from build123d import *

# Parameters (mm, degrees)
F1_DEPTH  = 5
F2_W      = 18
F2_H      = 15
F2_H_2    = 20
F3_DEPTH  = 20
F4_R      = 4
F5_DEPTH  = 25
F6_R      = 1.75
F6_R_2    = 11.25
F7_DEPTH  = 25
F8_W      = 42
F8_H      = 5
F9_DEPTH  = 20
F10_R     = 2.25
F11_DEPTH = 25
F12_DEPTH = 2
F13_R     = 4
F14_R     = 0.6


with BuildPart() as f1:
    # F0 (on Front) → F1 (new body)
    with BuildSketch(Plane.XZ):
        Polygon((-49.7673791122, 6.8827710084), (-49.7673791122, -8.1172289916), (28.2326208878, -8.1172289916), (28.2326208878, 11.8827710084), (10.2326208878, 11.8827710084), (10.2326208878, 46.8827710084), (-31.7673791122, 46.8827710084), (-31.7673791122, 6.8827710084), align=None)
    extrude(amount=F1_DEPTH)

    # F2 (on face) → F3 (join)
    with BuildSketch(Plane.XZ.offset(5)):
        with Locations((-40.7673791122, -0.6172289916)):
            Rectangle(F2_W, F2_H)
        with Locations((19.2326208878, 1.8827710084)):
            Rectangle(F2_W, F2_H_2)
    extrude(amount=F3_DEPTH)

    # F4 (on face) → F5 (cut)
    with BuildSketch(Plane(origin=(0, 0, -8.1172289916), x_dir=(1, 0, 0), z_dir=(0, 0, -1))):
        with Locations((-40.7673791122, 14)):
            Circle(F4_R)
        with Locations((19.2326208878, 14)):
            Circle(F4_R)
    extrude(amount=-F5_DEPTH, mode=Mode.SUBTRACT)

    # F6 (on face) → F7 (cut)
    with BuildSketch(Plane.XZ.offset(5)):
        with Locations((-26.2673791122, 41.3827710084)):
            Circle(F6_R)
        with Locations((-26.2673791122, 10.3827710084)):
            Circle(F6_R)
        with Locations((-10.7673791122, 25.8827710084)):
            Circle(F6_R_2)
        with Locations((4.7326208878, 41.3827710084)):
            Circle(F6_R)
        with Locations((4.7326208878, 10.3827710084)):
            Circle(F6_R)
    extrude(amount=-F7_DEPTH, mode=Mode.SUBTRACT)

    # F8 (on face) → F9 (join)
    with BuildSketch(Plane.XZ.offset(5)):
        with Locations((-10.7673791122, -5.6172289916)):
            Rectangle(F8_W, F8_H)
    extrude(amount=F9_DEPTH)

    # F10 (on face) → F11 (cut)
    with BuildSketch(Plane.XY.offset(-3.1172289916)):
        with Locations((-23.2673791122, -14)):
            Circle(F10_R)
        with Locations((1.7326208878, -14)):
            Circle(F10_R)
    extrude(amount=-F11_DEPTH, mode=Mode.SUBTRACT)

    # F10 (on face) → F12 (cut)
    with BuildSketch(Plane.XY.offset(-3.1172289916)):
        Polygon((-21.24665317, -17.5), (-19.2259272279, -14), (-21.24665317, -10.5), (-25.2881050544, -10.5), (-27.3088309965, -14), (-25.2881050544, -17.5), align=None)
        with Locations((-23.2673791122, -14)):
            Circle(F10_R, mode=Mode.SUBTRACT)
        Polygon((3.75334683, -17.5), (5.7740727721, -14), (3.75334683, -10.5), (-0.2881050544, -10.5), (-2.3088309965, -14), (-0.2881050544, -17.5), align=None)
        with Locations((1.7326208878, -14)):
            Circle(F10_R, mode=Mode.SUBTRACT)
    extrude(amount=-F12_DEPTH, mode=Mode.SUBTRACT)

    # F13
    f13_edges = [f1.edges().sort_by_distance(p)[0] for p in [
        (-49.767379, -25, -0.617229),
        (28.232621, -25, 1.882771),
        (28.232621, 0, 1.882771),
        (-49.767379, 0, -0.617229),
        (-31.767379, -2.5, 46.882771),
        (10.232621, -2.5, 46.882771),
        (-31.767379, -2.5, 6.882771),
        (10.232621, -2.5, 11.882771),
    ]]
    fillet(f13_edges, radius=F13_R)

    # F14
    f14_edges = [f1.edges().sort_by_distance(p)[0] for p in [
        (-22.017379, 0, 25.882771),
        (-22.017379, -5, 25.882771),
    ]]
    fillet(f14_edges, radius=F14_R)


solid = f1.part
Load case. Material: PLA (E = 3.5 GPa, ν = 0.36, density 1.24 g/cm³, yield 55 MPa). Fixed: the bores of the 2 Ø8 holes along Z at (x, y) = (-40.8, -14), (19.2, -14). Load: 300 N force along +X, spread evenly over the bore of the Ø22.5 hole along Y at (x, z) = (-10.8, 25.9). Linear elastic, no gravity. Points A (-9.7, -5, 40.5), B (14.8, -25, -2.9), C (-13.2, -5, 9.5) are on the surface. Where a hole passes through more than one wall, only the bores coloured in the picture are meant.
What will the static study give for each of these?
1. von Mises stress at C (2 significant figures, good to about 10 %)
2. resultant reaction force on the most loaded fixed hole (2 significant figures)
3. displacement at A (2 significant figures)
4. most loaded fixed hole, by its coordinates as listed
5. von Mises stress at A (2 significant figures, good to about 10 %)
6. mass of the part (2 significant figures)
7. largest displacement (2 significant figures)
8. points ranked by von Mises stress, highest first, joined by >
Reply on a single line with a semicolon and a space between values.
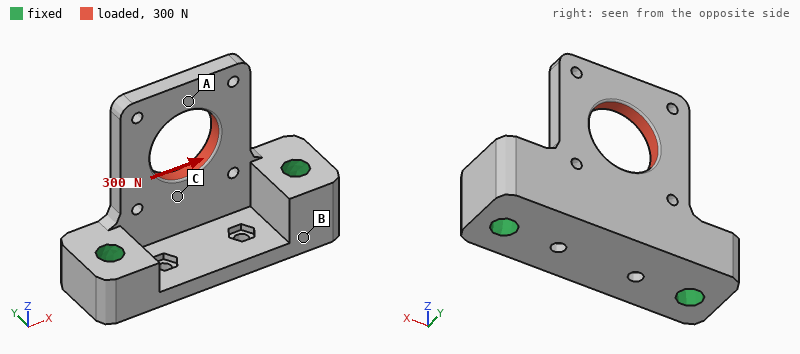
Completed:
3.7 MPa; 230 N; 0.13 mm; (19.2, -14); 2.1 MPa; 34 g; 0.15 mm; C > A > B
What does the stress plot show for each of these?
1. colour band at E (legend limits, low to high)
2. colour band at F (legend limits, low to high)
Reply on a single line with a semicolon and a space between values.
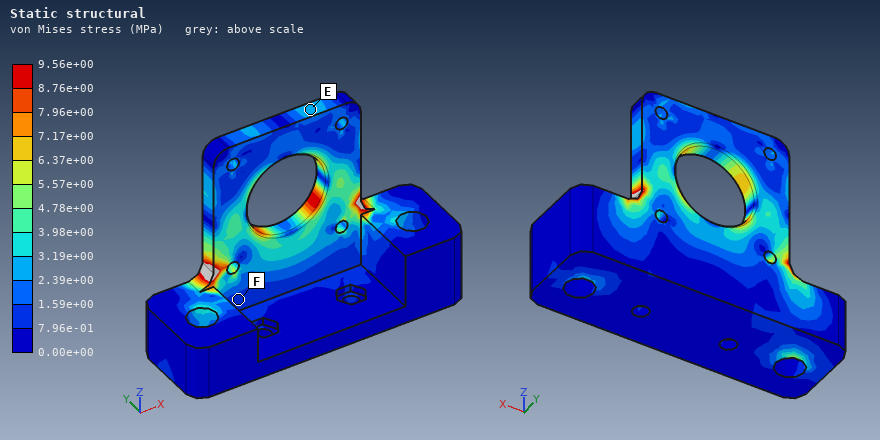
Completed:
2.39e+00 to 3.19e+00 MPa; 7.96e-01 to 1.59e+00 MPa
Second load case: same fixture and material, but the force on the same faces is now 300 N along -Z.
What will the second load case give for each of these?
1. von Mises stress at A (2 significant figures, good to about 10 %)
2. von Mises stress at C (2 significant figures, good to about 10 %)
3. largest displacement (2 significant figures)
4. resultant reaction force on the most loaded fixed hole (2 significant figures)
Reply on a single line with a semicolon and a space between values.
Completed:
0.89 MPa; 1.1 MPa; 63 µm; 160 N
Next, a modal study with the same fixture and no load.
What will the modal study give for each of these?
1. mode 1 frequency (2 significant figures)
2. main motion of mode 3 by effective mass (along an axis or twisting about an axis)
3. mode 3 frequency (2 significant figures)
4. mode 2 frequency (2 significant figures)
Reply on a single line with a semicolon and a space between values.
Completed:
630 Hz; along X; 2800 Hz; 1600 Hz
